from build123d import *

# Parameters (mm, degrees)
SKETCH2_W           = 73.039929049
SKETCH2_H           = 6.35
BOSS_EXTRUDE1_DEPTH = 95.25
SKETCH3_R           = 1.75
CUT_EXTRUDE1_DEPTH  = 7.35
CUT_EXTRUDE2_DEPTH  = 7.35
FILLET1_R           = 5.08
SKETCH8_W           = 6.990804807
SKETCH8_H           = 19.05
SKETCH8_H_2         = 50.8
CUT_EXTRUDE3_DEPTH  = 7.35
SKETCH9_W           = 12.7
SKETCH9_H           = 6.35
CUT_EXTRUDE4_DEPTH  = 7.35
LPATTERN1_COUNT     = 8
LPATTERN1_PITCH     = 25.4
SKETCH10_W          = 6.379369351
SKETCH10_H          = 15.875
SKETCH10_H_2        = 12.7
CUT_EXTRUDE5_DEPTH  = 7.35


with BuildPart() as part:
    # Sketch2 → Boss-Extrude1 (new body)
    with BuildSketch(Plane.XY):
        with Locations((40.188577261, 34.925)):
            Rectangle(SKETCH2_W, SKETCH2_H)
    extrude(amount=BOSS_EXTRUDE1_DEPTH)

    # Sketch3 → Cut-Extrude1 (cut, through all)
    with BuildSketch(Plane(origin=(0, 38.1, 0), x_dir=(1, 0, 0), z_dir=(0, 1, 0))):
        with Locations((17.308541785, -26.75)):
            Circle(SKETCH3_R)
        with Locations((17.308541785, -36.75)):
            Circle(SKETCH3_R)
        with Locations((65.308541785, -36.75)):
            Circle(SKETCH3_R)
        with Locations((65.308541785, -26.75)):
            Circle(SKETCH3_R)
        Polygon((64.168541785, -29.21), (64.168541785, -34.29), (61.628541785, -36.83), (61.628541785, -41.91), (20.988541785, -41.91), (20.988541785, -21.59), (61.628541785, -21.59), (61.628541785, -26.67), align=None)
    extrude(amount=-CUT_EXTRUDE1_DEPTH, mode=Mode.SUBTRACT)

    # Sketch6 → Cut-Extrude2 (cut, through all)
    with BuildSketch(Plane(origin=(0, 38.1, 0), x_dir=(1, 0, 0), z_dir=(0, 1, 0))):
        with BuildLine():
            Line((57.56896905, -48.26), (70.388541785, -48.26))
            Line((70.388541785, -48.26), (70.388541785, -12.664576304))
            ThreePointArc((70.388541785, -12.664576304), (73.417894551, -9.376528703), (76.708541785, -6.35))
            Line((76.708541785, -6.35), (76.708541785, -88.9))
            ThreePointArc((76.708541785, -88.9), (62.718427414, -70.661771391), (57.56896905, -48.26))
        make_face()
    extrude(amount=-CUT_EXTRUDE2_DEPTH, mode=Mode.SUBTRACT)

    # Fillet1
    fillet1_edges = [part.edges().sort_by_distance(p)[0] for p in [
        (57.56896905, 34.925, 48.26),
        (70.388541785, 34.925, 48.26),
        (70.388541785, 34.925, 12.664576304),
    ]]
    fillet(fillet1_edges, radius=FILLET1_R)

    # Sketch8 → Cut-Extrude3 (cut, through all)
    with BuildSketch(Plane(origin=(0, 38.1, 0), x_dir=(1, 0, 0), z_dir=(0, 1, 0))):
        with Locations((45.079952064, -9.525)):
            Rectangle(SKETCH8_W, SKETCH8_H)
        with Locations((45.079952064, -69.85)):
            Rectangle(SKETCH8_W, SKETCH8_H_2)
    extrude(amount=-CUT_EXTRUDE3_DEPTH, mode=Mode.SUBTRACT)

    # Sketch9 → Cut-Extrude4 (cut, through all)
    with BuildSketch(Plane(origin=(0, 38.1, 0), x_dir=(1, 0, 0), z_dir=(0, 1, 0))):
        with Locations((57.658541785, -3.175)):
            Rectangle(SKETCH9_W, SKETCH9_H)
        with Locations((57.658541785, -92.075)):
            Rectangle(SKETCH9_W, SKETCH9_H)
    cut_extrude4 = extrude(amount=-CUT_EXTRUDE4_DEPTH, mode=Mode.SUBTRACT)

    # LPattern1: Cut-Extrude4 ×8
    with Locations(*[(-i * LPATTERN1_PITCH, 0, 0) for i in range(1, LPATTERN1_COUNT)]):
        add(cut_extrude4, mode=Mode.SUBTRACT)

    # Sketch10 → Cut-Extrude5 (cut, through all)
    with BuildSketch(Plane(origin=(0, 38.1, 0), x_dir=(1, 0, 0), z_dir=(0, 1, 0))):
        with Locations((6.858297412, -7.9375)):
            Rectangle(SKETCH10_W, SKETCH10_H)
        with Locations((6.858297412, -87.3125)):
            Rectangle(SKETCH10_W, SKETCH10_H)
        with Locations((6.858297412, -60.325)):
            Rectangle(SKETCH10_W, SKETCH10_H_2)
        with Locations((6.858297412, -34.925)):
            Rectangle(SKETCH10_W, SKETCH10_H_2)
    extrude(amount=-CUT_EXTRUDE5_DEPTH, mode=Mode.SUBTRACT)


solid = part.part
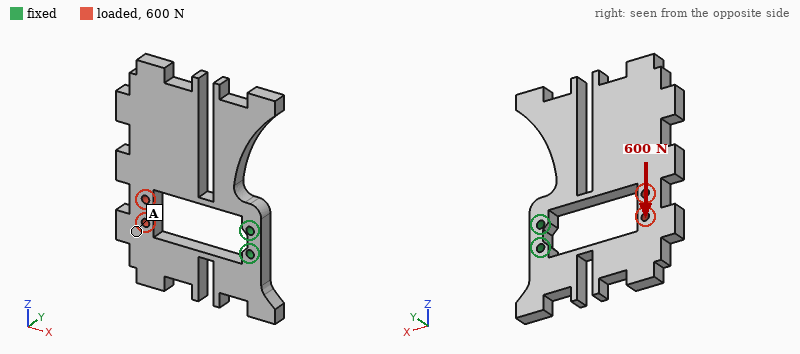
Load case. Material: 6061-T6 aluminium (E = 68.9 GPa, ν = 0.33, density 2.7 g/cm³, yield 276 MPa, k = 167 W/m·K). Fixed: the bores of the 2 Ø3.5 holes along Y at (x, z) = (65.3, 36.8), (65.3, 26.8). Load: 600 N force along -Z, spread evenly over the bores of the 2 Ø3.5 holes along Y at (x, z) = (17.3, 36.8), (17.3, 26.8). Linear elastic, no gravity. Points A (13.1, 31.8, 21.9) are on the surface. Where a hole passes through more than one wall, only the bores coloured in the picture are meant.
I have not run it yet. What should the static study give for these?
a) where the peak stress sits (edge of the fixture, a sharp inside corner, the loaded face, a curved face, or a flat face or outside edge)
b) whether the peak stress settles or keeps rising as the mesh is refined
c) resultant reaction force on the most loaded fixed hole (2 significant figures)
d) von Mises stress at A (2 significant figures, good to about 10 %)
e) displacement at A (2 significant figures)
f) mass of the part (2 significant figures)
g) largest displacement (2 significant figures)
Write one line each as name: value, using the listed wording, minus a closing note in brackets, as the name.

where the peak stress sits: edge of the fixture
whether the peak stress settles or keeps rising as the mesh is refined: keeps rising
resultant reaction force on the most loaded fixed hole: 1.3 kN
von Mises stress at A: 22 MPa
displacement at A: 0.31 mm
mass of the part: 70 g
largest displacement: 0.43 mm
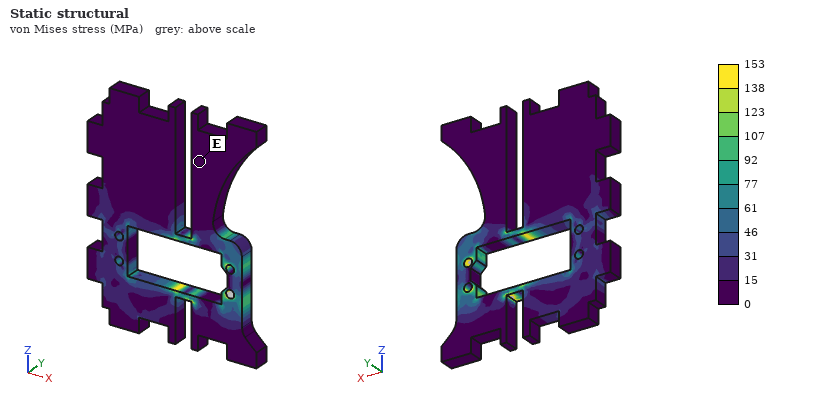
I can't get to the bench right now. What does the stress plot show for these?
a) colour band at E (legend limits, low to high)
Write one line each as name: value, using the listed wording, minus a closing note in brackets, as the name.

colour band at E: 0 to 15 MPa
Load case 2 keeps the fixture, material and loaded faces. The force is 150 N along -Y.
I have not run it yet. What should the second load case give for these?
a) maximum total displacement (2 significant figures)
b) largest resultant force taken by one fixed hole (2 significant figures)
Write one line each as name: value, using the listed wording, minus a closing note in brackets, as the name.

maximum total displacement: 0.63 mm
largest resultant force taken by one fixed hole: 77 N
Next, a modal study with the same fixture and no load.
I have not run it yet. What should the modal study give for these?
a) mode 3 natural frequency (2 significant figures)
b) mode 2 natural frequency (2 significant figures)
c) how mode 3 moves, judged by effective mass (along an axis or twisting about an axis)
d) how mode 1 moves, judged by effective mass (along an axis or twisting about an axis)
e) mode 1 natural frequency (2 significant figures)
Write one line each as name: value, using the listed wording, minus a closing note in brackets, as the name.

mode 3 natural frequency: 930 Hz
mode 2 natural frequency: 680 Hz
how mode 3 moves, judged by effective mass: along Y
how mode 1 moves, judged by effective mass: along Y
mode 1 natural frequency: 350 Hz
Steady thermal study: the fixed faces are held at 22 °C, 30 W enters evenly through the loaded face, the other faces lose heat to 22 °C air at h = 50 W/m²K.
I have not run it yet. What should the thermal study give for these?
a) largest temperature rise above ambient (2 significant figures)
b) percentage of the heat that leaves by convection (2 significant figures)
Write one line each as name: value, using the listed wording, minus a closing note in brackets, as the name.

largest temperature rise above ambient: 65 K
percentage of the heat that leaves by convection: 62 %
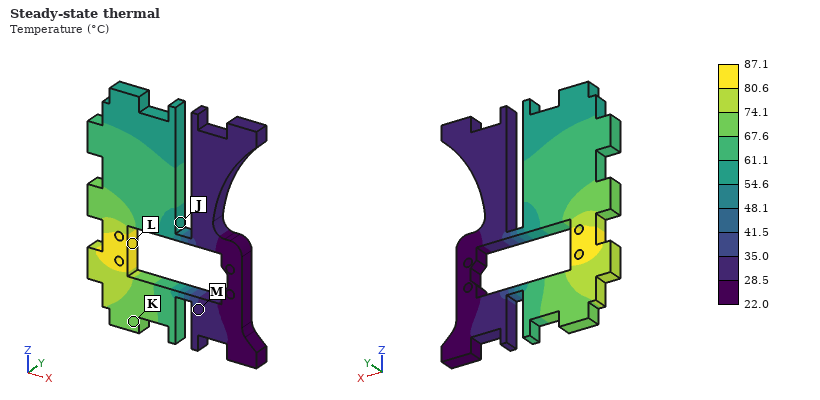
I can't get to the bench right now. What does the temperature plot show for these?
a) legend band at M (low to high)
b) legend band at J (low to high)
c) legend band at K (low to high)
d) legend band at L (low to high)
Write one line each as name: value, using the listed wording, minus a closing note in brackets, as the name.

legend band at M: 28.5 to 35.0 °C
legend band at J: 54.6 to 61.1 °C
legend band at K: 67.6 to 74.1 °C
legend band at L: 80.6 to 87.1 °C
